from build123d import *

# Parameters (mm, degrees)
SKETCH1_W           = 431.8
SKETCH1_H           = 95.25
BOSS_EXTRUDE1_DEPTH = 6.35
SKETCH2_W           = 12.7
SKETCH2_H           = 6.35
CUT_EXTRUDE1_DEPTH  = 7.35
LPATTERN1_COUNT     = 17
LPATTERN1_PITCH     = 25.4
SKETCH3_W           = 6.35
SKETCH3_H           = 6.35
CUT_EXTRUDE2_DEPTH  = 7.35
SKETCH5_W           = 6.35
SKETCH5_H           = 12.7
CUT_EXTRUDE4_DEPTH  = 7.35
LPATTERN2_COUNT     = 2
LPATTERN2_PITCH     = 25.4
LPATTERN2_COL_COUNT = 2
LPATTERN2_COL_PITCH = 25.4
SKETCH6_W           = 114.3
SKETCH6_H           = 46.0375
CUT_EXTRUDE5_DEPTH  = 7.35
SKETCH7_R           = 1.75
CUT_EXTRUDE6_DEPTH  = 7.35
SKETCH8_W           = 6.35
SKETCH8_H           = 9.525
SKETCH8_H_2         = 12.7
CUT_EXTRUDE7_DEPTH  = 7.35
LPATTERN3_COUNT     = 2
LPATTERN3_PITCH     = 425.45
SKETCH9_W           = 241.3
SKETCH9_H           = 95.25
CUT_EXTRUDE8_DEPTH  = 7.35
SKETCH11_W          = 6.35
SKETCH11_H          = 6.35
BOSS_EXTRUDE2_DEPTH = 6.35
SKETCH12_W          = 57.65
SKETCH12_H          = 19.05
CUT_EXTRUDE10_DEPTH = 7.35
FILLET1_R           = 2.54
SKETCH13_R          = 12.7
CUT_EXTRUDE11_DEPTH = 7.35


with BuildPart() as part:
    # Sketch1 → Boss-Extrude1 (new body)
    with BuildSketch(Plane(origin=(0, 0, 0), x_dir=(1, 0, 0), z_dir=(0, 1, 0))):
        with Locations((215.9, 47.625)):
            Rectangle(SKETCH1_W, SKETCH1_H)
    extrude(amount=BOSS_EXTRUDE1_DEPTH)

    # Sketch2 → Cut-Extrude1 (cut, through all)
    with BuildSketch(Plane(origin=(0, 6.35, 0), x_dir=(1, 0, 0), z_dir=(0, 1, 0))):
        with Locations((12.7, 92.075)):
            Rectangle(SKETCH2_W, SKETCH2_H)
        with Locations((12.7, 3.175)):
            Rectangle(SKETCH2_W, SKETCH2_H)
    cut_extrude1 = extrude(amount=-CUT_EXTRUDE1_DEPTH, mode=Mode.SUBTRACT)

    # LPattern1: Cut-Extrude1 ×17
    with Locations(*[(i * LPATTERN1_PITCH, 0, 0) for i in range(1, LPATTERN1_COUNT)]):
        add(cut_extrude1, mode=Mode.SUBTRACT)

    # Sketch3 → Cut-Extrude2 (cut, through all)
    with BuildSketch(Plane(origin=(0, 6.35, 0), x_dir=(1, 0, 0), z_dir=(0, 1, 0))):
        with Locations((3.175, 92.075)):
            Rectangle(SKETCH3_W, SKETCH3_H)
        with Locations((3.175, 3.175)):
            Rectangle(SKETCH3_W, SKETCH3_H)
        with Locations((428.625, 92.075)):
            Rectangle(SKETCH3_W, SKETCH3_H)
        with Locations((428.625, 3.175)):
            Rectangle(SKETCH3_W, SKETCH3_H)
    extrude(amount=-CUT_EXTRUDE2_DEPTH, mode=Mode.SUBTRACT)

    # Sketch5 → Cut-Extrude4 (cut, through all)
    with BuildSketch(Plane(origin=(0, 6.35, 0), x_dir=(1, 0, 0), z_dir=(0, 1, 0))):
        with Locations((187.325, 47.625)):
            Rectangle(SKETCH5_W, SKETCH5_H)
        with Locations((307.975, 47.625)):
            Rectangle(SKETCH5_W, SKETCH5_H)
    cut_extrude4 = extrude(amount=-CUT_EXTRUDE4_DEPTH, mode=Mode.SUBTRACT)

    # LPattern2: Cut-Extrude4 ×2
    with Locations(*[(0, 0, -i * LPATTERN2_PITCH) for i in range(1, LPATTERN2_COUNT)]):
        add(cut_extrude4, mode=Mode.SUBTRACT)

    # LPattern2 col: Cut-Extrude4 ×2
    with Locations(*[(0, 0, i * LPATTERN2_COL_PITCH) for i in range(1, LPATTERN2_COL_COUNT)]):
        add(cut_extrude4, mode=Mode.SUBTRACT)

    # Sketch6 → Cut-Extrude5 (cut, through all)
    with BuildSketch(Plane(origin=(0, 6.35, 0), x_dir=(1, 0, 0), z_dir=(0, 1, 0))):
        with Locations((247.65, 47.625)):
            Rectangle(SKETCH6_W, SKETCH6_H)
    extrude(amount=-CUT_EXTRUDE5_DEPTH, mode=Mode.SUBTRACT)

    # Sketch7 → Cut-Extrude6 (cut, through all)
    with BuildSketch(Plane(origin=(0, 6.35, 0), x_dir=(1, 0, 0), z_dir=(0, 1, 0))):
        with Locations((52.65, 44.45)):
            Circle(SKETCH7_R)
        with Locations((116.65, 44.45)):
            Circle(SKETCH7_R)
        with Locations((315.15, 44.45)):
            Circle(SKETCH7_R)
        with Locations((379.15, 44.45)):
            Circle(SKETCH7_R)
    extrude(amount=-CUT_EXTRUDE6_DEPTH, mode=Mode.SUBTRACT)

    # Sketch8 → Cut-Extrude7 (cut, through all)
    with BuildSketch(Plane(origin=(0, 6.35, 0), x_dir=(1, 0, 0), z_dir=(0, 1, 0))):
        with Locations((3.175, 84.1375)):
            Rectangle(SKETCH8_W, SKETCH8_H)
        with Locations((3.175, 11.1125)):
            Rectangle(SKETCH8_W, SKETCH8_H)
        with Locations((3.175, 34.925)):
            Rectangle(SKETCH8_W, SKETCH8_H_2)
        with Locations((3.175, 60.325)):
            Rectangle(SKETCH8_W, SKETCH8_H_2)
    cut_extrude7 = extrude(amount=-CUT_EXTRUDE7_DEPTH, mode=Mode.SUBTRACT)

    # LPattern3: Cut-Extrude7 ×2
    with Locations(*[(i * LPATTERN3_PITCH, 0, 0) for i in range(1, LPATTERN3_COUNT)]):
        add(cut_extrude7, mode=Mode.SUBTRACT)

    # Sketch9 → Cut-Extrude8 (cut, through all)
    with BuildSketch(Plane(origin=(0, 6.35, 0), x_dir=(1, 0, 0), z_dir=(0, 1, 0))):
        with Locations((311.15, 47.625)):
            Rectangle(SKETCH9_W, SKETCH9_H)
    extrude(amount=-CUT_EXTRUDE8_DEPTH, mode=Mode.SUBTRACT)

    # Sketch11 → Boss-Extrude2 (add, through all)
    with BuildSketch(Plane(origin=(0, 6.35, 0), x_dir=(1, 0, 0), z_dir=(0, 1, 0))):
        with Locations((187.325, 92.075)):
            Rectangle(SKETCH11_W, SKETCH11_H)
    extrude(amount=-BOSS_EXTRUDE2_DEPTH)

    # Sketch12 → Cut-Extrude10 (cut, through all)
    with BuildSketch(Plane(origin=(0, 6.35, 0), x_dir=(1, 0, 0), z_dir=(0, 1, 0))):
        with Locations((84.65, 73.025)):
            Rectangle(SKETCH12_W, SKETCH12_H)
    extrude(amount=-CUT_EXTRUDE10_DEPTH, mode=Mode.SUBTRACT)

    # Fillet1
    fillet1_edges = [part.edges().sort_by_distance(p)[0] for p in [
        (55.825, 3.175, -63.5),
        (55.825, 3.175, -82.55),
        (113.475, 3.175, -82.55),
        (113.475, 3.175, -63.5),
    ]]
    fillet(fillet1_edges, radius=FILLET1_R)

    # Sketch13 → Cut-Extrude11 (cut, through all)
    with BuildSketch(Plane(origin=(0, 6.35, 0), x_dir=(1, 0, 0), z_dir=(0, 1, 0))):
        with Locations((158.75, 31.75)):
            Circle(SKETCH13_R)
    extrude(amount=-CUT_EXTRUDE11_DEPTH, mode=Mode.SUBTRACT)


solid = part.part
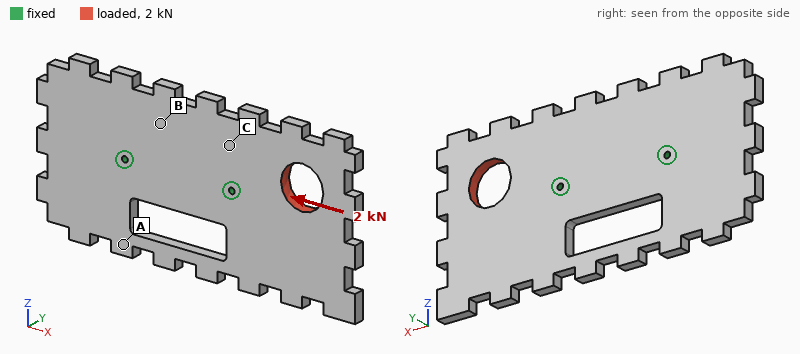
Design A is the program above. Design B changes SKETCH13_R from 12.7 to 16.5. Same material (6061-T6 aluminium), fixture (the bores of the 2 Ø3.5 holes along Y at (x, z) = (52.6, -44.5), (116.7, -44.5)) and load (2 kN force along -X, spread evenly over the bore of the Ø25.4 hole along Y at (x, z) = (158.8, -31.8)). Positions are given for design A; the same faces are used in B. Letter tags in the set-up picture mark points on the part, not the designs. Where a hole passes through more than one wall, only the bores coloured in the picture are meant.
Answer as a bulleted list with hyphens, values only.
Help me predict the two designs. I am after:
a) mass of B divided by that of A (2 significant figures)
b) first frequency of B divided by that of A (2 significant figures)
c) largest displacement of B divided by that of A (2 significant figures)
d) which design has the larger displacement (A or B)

- 0.98
- 0.99
- 1.3
- B
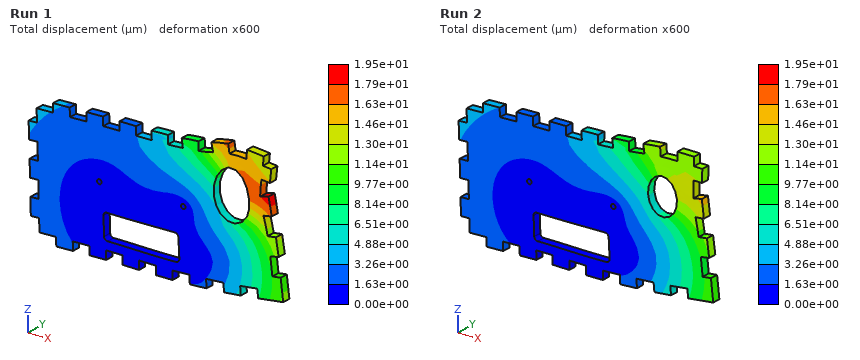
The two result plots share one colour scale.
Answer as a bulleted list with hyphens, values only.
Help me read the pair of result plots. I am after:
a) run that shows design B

- Run 1
